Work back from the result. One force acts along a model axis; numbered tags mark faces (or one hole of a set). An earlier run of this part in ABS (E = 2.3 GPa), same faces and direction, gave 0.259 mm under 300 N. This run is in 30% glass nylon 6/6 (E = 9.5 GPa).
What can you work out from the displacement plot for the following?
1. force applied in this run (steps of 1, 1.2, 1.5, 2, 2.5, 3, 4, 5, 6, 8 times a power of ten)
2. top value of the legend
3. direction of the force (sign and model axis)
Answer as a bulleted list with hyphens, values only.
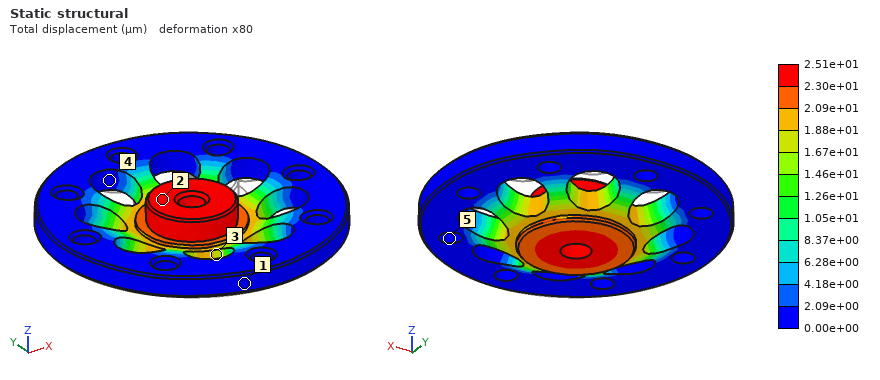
- 120 N
- 2.51e+01 µm
- -Z
